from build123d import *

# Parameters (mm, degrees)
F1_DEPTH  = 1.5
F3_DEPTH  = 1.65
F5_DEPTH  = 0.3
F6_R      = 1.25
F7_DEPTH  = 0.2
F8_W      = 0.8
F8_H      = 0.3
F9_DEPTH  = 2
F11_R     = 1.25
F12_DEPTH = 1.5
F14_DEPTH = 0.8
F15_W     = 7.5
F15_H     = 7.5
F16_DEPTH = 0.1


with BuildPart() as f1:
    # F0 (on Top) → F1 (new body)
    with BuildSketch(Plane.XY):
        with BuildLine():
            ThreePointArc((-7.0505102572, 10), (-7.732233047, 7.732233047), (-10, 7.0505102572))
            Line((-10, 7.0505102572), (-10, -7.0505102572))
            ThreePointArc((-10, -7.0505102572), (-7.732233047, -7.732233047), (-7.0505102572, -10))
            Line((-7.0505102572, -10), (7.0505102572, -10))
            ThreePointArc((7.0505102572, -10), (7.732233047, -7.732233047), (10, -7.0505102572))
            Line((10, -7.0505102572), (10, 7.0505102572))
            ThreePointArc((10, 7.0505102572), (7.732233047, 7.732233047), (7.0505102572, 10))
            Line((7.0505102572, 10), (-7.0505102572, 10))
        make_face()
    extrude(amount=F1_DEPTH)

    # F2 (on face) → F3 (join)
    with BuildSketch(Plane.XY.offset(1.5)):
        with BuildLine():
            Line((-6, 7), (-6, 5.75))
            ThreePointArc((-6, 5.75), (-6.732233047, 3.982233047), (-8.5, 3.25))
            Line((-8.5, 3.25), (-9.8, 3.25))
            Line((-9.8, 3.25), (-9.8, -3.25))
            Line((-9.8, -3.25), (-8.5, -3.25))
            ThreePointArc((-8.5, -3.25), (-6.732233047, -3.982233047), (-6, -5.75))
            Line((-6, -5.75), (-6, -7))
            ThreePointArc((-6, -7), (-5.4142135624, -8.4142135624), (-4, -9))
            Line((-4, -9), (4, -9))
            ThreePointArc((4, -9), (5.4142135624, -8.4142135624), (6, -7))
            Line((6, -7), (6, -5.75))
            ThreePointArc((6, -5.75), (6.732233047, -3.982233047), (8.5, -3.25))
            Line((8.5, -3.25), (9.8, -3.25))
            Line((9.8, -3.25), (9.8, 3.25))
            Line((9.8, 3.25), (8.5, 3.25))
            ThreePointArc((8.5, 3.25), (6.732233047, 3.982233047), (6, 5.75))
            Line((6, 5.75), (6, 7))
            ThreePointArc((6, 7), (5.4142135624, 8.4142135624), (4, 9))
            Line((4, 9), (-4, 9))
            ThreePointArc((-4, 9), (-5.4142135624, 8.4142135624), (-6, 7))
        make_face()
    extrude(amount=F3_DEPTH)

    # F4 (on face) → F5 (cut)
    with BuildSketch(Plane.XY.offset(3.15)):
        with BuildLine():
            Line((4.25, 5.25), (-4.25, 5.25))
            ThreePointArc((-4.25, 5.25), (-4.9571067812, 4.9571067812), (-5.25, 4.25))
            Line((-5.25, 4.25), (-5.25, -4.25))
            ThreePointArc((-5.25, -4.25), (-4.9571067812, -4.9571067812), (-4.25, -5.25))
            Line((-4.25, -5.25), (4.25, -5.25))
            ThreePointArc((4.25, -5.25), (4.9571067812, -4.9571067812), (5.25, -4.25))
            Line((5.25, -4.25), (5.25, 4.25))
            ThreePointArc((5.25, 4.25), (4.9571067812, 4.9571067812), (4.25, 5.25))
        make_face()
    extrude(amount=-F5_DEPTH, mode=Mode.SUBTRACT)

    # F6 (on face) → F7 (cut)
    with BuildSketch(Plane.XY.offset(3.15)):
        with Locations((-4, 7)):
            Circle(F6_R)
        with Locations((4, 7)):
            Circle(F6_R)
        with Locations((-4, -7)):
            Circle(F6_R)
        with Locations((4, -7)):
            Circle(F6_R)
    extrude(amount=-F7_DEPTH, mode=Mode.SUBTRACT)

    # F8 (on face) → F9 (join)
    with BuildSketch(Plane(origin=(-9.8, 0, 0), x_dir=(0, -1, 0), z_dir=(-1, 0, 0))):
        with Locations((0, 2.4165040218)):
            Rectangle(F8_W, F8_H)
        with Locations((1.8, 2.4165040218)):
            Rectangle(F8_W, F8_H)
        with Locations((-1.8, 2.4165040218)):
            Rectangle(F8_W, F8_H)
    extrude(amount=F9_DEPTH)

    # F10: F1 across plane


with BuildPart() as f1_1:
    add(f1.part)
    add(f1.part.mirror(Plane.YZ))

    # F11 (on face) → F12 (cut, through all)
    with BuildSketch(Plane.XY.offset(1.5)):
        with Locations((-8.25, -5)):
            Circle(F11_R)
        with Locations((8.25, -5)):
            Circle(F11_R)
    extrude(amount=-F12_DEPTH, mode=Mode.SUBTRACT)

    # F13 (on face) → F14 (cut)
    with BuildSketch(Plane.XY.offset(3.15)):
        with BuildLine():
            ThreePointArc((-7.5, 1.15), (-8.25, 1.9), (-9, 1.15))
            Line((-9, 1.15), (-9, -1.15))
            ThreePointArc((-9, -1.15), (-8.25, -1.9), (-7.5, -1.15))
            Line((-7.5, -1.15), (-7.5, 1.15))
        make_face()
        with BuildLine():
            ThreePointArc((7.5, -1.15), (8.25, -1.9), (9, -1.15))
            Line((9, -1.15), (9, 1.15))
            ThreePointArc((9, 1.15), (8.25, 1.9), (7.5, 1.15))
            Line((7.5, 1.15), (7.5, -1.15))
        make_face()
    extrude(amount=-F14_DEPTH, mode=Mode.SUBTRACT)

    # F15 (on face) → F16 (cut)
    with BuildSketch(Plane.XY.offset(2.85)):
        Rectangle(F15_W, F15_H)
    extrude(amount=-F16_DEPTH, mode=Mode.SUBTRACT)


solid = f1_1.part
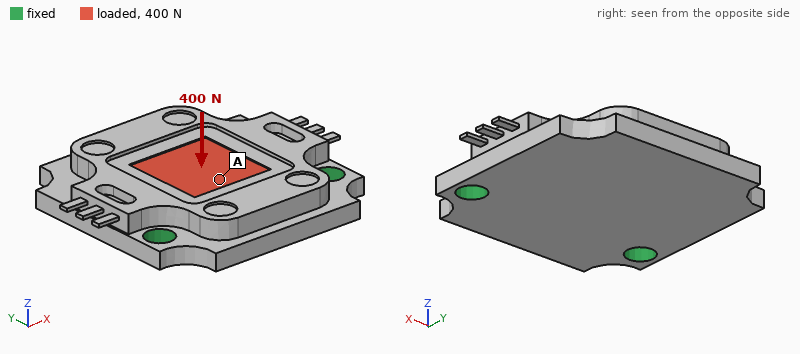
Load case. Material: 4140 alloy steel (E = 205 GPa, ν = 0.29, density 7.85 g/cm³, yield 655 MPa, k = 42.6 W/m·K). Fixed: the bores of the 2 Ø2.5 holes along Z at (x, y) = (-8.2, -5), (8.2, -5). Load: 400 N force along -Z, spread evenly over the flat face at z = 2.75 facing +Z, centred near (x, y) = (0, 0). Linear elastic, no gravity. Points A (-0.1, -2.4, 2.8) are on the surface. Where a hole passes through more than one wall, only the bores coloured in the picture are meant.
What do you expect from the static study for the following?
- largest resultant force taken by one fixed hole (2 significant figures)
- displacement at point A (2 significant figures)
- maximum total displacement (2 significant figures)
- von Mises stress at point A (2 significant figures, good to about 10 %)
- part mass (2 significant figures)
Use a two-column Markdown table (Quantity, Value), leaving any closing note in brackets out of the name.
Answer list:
| Quantity | Value |
|---|---|
| largest resultant force taken by one fixed hole | 260 N |
| displacement at point A | 9.0 µm |
| maximum total displacement | 38 µm |
| von Mises stress at point A | 53 MPa |
| part mass | 7.3 g |
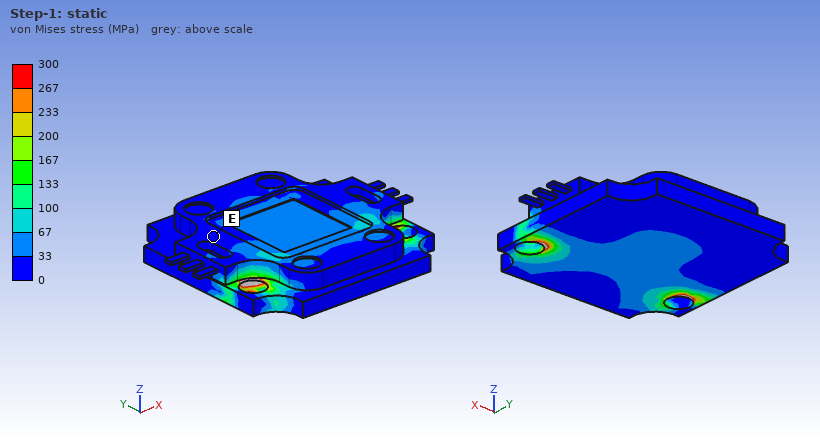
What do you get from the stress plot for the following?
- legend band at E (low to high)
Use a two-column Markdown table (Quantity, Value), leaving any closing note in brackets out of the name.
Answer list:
| Quantity | Value |
|---|---|
| legend band at E | 0 to 33 MPa |
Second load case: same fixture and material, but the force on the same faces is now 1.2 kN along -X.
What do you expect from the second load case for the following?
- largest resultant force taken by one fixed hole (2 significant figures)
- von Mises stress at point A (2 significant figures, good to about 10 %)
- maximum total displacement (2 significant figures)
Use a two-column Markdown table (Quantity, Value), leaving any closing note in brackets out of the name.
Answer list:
| Quantity | Value |
|---|---|
| largest resultant force taken by one fixed hole | 710 N |
| von Mises stress at point A | 57 MPa |
| maximum total displacement | 3.5 µm |
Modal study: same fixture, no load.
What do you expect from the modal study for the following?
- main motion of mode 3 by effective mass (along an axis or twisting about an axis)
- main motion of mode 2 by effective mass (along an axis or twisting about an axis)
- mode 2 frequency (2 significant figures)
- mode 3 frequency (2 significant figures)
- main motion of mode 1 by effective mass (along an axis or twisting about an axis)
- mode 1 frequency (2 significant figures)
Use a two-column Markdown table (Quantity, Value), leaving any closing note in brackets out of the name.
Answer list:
| Quantity | Value |
|---|---|
| main motion of mode 3 by effective mass | along Z |
| main motion of mode 2 by effective mass | twisting about Y |
| mode 2 frequency | 23 kHz |
| mode 3 frequency | 36 kHz |
| main motion of mode 1 by effective mass | along Z |
| mode 1 frequency | 7200 Hz |
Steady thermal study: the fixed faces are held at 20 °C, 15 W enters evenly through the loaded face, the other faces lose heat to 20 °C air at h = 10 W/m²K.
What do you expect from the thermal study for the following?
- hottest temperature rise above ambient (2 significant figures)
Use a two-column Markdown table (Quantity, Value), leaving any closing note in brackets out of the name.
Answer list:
| Quantity | Value |
|---|---|
| hottest temperature rise above ambient | 68 K |
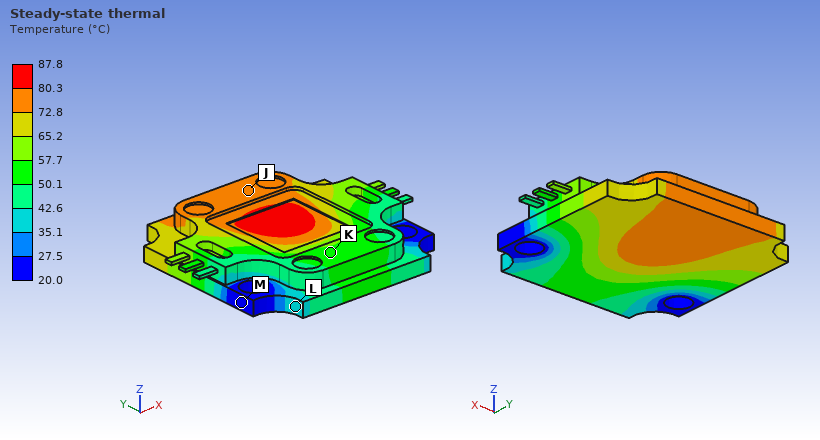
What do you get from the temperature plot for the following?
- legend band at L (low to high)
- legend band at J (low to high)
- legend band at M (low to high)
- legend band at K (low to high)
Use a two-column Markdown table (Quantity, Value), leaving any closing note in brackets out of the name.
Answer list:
| Quantity | Value |
|---|---|
| legend band at L | 35.1 to 42.6 °C |
| legend band at J | 72.8 to 80.3 °C |
| legend band at M | 20.0 to 27.5 °C |
| legend band at K | 50.1 to 57.7 °C |
